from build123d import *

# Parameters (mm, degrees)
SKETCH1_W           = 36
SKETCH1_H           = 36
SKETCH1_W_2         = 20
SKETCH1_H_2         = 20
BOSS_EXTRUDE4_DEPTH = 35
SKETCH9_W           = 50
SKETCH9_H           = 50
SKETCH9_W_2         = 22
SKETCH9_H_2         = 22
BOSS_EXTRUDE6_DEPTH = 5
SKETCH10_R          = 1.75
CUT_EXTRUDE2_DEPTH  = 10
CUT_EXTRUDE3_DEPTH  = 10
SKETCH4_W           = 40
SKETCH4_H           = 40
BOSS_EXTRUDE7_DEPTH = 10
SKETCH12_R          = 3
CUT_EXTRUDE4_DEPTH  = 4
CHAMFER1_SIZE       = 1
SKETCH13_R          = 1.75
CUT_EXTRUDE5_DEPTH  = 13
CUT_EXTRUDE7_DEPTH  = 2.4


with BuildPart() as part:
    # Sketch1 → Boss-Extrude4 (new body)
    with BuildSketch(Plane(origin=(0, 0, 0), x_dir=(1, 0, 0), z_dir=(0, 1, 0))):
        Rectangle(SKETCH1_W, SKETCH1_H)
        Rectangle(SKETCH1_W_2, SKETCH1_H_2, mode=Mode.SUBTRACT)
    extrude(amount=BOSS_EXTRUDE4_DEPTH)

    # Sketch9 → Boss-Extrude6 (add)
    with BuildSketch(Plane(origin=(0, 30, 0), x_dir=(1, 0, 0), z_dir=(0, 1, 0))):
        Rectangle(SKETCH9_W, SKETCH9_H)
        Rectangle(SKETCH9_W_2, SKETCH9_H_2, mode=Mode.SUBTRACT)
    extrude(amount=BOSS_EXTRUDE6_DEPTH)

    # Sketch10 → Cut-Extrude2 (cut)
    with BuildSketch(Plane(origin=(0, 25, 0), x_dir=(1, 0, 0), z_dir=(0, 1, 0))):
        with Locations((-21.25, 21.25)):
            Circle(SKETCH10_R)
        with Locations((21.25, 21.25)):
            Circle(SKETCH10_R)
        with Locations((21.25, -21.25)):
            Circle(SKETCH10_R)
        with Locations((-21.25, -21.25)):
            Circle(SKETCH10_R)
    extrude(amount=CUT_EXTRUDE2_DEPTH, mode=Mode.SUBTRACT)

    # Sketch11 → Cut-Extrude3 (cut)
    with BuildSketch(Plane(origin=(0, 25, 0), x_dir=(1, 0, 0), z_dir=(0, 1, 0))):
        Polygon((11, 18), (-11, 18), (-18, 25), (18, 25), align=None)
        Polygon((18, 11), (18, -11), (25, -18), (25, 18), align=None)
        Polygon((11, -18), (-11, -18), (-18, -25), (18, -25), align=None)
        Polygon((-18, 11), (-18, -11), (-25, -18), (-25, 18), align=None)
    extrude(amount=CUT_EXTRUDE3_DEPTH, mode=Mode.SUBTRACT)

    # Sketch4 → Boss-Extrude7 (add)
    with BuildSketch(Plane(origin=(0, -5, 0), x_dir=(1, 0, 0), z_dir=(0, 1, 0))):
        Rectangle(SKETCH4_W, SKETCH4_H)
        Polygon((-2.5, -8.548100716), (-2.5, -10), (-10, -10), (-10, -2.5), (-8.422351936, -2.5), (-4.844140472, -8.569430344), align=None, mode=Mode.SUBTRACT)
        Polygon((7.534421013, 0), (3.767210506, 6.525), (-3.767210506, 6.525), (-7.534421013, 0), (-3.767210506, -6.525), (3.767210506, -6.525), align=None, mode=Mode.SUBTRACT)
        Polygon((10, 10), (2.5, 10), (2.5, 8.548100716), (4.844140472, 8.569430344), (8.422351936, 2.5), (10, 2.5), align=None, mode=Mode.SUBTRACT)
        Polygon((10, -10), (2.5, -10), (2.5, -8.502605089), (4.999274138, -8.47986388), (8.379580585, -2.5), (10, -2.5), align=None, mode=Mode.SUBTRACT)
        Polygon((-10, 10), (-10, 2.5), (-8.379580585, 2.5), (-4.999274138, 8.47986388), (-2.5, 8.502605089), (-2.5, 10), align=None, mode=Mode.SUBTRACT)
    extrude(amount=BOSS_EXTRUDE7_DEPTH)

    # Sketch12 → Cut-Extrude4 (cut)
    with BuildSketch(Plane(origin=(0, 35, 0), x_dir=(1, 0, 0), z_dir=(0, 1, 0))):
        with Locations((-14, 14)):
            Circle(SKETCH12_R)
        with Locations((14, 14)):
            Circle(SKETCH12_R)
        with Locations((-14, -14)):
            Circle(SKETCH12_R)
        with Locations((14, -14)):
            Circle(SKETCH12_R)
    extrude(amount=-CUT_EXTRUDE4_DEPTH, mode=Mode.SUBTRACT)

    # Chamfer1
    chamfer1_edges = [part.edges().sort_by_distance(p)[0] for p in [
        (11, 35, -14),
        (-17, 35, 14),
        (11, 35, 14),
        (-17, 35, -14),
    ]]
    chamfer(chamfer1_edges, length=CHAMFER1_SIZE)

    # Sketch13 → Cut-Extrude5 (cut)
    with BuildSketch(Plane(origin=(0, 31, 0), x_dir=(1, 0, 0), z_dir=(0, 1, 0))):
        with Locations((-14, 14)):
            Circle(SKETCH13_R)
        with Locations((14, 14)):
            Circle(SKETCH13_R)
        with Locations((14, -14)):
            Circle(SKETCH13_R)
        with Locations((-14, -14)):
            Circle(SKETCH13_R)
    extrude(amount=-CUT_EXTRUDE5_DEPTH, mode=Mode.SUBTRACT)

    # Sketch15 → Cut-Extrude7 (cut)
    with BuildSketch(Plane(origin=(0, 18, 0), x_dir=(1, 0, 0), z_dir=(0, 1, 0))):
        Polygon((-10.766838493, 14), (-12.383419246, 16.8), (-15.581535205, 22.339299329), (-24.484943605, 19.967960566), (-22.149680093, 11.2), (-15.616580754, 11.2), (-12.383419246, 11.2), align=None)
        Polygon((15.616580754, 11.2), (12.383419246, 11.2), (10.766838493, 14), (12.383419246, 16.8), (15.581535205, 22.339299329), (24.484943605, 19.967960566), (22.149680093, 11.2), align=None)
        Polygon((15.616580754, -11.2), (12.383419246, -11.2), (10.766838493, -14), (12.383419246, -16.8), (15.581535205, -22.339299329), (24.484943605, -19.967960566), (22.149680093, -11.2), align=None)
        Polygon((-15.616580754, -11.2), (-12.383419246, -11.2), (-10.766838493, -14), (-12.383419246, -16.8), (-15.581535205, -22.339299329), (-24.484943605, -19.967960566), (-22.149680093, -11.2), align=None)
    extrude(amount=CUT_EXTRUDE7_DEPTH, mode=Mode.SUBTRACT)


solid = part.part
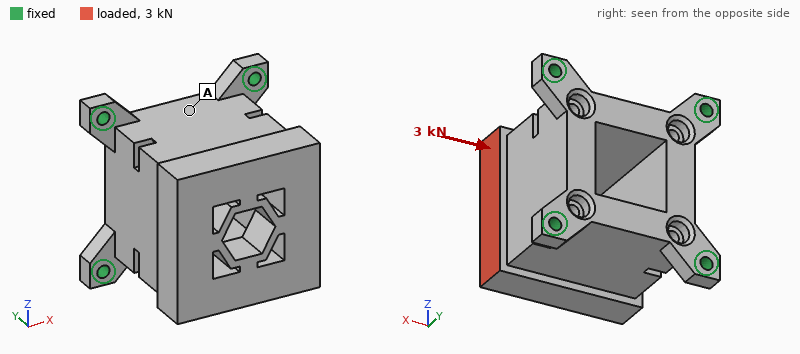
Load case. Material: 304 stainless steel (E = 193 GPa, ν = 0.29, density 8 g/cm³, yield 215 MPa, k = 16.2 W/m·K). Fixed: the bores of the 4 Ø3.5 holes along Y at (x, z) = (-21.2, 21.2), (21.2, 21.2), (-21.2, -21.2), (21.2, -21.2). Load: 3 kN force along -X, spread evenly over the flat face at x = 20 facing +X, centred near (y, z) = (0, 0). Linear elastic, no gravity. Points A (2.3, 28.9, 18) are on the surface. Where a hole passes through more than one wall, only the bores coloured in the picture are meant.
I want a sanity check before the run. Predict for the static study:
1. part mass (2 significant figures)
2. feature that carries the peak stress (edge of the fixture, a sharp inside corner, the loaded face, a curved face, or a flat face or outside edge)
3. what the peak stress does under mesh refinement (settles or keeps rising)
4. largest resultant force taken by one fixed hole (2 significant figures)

320 g
edge of the fixture
keeps rising
1.6 kN
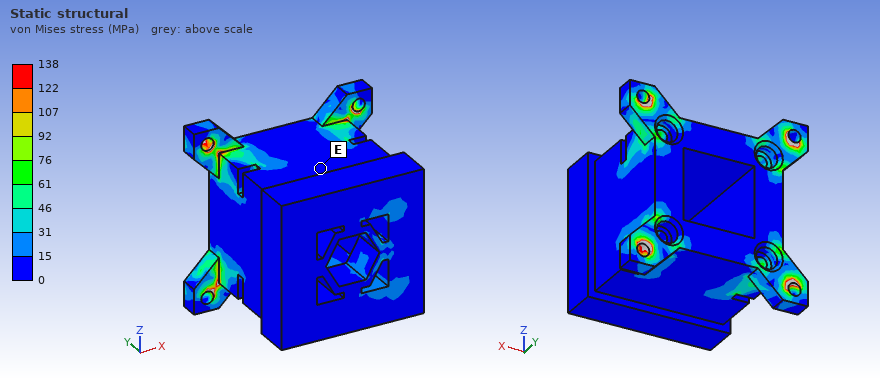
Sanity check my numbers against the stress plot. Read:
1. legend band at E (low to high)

0 to 15 MPa
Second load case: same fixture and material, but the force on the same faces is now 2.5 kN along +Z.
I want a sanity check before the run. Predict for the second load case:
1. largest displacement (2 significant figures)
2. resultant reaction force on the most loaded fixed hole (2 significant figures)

24 µm
1.5 kN
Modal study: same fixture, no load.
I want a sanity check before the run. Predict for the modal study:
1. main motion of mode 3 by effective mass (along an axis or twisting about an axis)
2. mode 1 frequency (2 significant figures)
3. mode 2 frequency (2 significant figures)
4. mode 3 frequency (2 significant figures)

along Y
4800 Hz
4900 Hz
7100 Hz
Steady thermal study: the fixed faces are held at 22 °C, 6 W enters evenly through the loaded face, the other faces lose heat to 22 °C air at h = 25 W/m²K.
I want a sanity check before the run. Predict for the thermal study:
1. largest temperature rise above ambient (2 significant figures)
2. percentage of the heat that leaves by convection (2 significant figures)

27 K
64 %
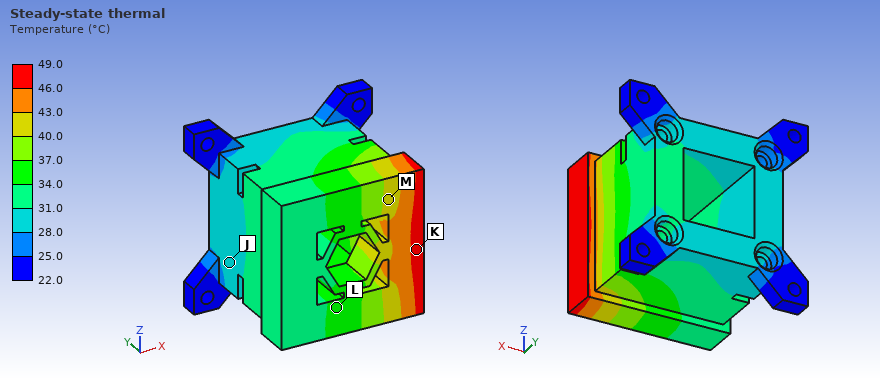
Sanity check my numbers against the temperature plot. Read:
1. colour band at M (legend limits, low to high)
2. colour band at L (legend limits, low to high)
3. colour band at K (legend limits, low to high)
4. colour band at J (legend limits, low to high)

40.0 to 43.0 °C
34.0 to 37.0 °C
46.0 to 49.0 °C
28.0 to 31.0 °C
